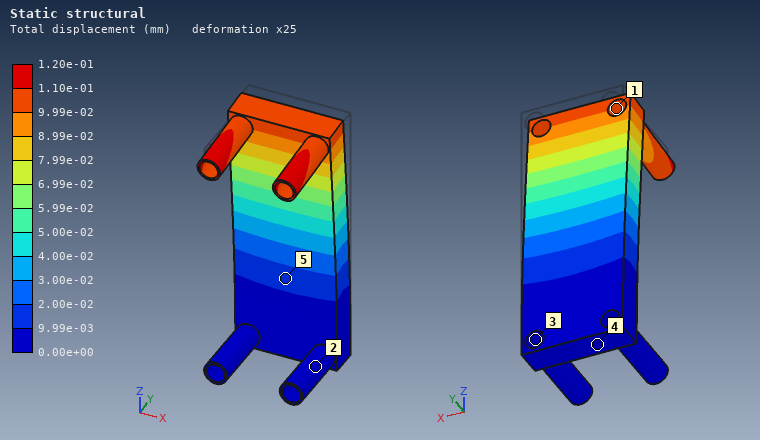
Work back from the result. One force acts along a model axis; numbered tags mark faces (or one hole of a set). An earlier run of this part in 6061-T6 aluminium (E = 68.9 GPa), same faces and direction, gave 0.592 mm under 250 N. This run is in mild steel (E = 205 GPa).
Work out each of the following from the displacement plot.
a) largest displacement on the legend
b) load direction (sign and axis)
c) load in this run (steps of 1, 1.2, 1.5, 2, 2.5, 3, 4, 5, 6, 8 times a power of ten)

1.20e-01 mm
-Y
150 N
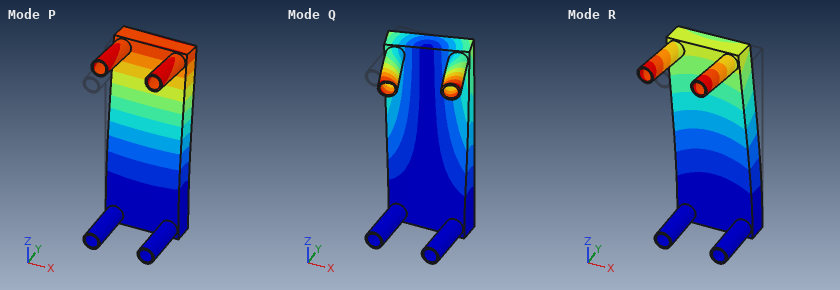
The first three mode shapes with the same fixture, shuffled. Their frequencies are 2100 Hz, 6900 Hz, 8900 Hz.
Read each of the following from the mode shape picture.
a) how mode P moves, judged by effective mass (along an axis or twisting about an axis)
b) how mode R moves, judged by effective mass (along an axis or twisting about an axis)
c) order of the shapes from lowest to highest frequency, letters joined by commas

along Y
along X
P, R, Q
